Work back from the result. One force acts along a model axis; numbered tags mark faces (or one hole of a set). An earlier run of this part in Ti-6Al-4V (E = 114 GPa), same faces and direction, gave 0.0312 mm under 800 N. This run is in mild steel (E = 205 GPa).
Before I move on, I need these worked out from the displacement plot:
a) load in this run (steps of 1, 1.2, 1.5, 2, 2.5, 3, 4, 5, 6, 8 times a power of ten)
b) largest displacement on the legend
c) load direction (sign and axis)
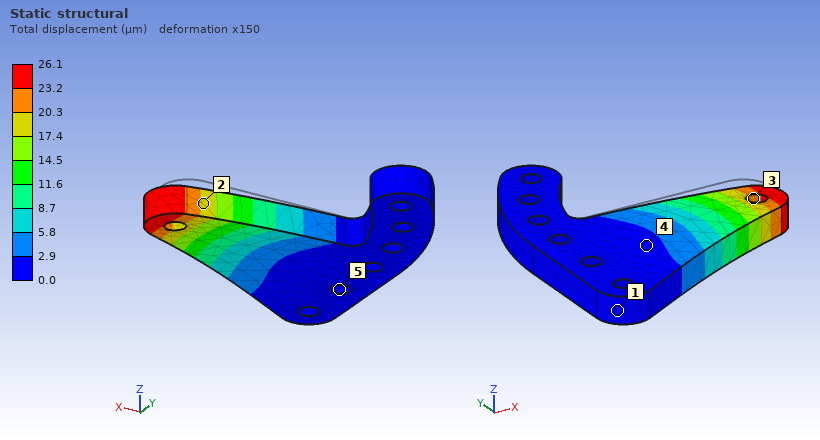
1.2 kN
26.1 µm
-Y
